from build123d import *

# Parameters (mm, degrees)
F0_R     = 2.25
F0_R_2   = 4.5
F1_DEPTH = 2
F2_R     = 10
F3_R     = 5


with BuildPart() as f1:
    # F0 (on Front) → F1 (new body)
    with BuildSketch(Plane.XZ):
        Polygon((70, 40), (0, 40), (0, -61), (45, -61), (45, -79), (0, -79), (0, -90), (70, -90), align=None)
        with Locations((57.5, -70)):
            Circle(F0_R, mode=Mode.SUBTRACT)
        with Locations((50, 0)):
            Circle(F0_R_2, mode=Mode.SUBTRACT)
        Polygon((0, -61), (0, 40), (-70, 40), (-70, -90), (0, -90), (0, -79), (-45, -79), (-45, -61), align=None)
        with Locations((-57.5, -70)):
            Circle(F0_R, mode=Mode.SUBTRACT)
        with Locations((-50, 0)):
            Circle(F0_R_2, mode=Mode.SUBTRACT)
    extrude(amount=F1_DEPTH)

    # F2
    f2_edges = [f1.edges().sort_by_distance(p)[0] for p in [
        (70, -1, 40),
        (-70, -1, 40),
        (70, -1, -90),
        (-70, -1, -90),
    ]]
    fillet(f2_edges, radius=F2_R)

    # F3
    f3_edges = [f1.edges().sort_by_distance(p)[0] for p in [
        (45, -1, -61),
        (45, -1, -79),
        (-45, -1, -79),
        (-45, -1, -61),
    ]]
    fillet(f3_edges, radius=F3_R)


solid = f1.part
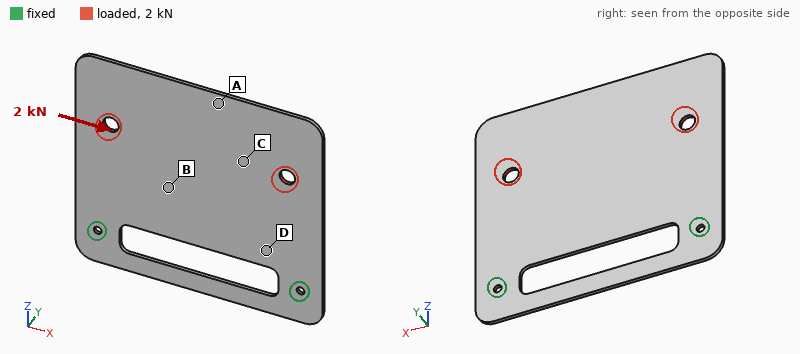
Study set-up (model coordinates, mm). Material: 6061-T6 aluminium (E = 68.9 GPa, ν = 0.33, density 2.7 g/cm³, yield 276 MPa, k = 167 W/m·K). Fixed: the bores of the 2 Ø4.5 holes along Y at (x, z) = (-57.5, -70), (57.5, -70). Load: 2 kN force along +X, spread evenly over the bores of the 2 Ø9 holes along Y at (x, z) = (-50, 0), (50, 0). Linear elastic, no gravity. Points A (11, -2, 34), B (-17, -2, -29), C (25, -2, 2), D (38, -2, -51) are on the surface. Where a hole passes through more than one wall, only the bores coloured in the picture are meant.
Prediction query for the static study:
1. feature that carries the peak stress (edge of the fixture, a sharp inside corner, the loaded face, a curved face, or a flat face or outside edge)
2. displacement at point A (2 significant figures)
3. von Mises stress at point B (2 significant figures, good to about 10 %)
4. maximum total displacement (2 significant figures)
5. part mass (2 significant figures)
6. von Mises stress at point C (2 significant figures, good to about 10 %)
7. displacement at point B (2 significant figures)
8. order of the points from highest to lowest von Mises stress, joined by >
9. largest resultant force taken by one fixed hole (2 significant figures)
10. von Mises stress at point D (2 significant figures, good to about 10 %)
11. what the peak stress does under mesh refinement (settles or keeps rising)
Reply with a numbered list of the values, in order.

1. edge of the fixture
2. 58 µm
3. 19 MPa
4. 60 µm
5. 88 g
6. 12 MPa
7. 37 µm
8. D > B > C > A
9. 1.5 kN
10. 29 MPa
11. keeps rising
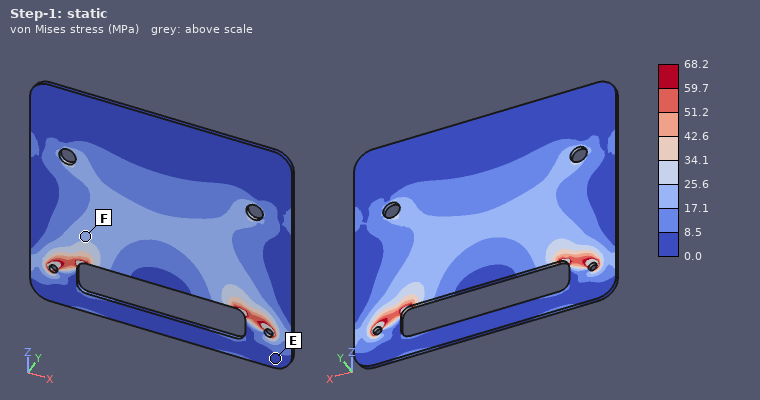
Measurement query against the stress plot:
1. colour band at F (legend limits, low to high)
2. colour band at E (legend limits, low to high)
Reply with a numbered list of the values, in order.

1. 17.1 to 25.6 MPa
2. 0.0 to 8.5 MPa
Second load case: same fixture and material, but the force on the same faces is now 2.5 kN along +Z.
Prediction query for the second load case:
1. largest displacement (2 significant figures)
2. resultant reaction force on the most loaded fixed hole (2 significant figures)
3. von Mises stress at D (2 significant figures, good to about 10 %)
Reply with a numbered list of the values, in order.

1. 24 µm
2. 1.3 kN
3. 13 MPa
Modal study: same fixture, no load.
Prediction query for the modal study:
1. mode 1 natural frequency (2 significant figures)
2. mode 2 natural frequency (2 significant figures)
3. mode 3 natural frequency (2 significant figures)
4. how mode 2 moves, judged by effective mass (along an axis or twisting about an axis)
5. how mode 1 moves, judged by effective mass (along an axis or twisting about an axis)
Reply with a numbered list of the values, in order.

1. 97 Hz
2. 280 Hz
3. 610 Hz
4. twisting about Z
5. along Y
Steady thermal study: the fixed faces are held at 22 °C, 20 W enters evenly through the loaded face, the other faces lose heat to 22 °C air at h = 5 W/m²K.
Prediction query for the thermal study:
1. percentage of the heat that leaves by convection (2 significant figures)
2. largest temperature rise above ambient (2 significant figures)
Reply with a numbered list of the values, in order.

1. 24 %
2. 47 K
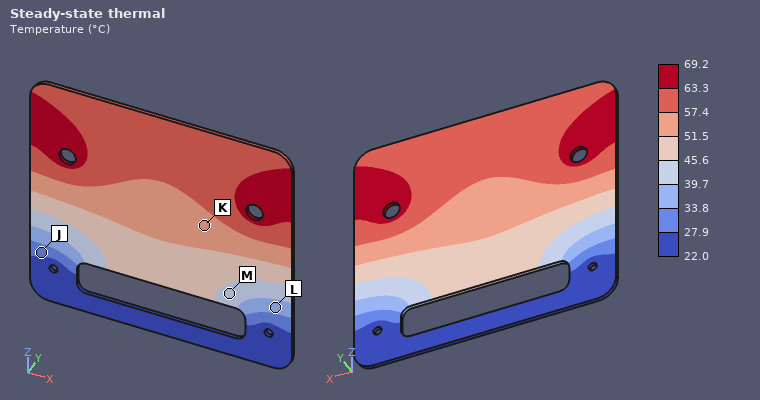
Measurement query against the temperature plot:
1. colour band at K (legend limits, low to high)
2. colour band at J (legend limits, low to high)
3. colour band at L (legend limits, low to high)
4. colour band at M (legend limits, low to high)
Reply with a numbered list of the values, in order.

1. 51.5 to 57.4 °C
2. 27.9 to 33.8 °C
3. 33.8 to 39.7 °C
4. 39.7 to 45.6 °C
